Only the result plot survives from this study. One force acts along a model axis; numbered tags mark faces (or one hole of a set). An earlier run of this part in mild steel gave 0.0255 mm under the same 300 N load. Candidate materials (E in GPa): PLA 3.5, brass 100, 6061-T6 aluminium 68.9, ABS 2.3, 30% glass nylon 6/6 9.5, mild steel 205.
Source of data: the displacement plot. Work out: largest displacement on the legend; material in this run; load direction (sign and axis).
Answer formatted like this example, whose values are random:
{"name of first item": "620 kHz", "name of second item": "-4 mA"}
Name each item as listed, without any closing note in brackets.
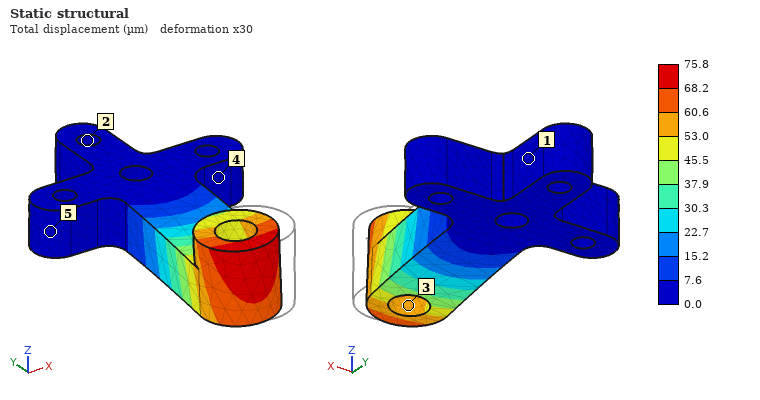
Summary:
{"largest displacement on the legend": "75.8 µm", "material in this run": "6061-T6 aluminium", "load direction": "-X"}
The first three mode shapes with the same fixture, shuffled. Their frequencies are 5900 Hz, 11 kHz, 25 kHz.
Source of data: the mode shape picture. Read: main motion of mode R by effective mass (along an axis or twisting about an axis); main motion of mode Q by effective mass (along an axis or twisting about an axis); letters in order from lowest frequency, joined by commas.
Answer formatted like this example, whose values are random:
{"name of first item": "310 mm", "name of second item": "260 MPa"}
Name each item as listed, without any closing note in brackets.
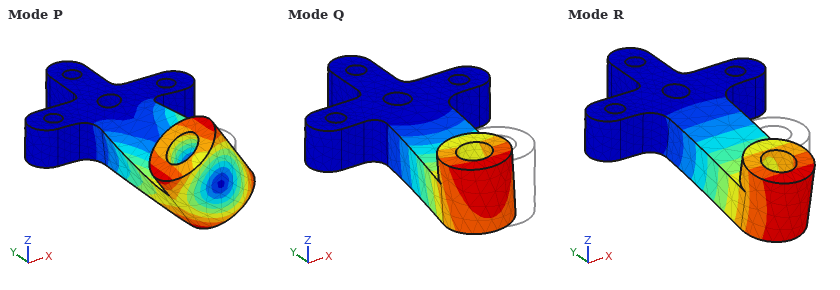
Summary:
{"main motion of mode R by effective mass": "along Z", "main motion of mode Q by effective mass": "along X", "letters in order from lowest frequency, joined by commas": "R, Q, P"}
